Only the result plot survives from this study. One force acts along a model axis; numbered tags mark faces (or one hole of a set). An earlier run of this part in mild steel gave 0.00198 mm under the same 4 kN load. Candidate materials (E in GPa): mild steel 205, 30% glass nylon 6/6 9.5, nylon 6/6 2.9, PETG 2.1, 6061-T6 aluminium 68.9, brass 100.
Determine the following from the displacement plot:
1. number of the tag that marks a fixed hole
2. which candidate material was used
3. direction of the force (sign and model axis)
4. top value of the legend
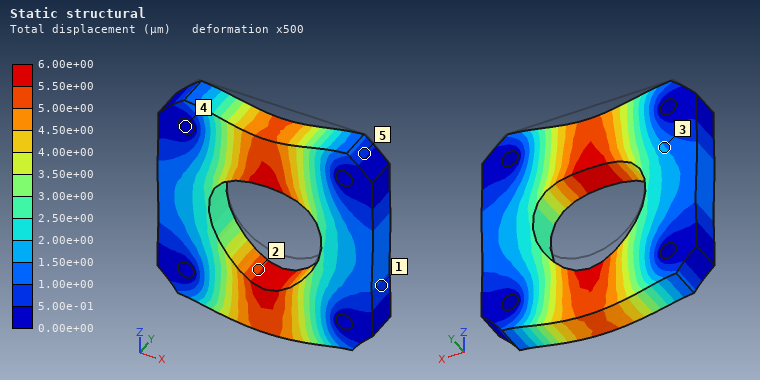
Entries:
4
6061-T6 aluminium
-Z
6.00e+00 µm
